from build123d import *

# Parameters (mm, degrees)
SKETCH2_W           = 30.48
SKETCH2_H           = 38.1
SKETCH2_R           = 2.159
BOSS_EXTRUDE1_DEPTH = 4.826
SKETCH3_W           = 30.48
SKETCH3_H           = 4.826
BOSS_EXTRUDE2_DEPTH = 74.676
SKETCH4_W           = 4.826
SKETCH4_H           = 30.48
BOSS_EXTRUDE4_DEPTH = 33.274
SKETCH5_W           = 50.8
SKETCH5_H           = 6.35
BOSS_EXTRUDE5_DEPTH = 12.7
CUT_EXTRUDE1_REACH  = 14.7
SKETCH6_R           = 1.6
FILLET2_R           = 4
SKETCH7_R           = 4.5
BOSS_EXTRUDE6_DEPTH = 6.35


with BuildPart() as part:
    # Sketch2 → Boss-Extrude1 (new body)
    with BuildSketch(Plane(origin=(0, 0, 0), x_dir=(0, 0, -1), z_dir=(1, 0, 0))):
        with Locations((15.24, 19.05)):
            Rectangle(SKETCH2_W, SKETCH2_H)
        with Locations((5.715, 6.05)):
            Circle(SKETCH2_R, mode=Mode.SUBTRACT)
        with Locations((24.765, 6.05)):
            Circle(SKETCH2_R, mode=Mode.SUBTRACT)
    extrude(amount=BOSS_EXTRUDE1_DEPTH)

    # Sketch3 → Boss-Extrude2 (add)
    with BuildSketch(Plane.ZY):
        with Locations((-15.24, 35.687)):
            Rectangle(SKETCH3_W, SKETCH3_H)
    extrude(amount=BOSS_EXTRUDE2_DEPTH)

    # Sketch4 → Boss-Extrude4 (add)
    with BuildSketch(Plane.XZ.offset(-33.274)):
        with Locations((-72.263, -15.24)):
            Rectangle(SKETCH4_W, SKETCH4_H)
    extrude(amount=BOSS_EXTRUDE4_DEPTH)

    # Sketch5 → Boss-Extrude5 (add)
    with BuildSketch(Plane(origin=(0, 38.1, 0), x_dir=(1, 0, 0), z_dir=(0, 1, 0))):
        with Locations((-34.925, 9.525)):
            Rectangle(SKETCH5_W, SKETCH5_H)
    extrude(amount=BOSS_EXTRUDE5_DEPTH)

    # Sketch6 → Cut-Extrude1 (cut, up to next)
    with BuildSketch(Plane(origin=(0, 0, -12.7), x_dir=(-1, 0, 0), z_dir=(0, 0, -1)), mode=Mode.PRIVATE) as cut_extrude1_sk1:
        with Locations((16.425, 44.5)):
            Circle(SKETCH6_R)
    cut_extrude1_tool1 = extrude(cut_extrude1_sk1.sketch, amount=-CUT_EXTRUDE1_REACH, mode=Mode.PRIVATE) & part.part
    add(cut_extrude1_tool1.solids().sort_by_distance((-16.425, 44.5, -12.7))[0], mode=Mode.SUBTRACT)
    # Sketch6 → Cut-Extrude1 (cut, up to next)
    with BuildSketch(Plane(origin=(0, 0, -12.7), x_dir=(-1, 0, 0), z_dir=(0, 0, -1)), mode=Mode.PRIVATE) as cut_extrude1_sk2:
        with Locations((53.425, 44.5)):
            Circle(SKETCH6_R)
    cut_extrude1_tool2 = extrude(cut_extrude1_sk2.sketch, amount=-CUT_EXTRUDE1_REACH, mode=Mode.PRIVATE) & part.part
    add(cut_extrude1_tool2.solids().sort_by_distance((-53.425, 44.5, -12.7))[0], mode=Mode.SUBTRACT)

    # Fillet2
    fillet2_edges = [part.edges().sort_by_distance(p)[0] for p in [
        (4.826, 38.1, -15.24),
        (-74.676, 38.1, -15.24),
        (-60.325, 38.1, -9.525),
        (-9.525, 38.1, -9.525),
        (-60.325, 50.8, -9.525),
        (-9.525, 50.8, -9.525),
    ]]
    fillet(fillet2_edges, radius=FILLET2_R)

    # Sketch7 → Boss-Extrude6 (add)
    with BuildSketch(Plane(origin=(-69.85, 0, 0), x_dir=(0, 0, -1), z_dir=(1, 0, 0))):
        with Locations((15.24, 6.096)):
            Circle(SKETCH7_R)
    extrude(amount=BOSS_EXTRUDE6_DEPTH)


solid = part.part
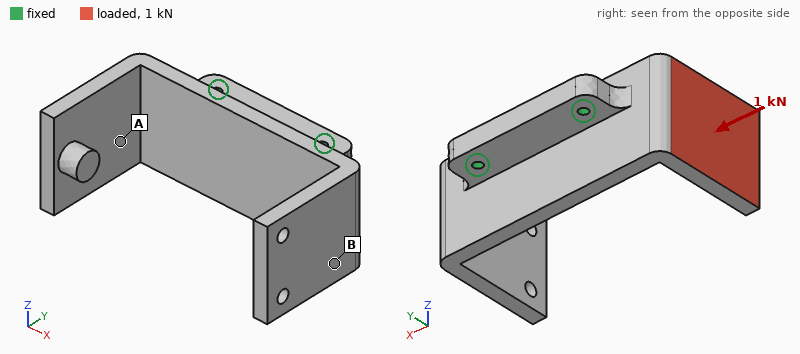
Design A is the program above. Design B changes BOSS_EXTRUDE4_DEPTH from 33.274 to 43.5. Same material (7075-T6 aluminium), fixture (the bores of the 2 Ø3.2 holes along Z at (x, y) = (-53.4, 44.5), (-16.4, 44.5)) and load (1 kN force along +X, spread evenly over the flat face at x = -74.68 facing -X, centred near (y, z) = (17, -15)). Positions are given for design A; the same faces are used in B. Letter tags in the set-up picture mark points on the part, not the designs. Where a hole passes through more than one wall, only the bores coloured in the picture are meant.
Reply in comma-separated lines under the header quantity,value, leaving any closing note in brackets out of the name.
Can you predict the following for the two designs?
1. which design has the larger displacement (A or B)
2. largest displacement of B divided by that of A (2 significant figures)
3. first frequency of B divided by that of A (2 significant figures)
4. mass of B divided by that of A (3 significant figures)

quantity,value
which design has the larger displacement,B
largest displacement of B divided by that of A,1.8
first frequency of B divided by that of A,0.72
mass of B divided by that of A,1.06
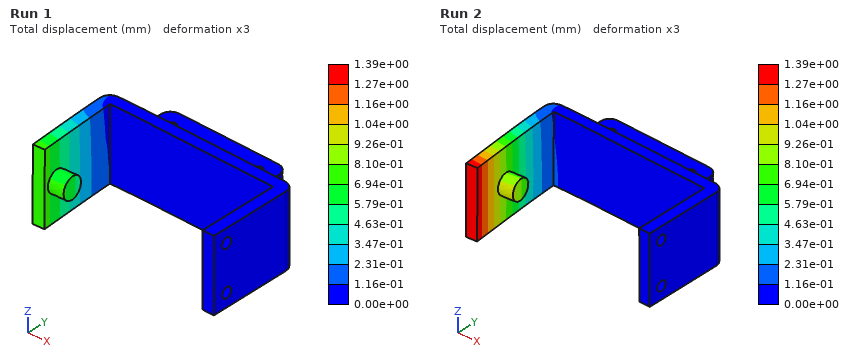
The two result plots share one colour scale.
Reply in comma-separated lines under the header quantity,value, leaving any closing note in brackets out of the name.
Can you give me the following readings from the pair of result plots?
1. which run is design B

quantity,value
which run is design B,Run 2
